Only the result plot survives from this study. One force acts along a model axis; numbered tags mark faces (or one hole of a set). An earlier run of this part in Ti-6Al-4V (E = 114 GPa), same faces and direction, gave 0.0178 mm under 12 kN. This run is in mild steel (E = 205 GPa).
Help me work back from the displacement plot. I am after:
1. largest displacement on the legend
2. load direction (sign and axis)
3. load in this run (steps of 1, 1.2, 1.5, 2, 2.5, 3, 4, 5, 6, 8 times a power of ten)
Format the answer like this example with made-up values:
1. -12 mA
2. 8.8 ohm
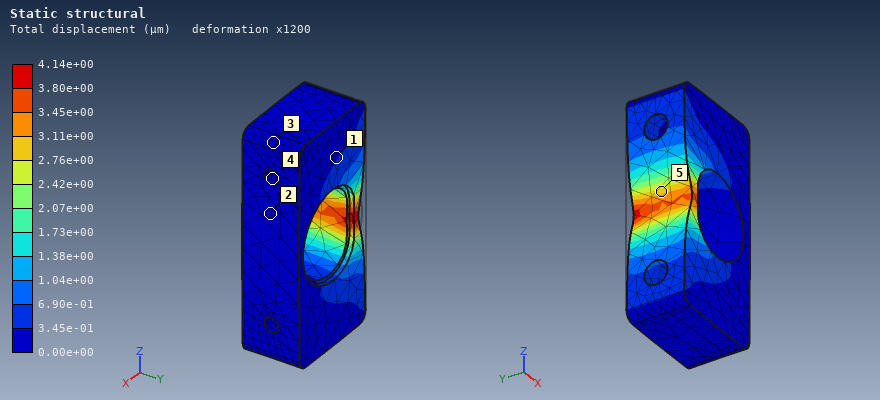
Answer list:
1. 4.14e+00 µm
2. +X
3. 5 kN
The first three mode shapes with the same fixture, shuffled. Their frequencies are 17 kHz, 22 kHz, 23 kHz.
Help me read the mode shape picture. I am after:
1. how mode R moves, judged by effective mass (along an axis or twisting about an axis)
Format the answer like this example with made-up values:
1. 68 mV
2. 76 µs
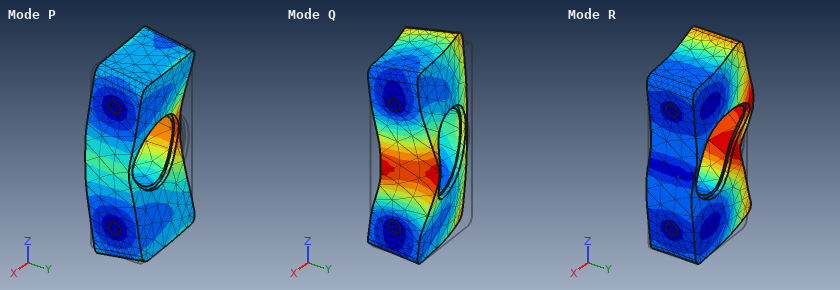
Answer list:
1. along Z
